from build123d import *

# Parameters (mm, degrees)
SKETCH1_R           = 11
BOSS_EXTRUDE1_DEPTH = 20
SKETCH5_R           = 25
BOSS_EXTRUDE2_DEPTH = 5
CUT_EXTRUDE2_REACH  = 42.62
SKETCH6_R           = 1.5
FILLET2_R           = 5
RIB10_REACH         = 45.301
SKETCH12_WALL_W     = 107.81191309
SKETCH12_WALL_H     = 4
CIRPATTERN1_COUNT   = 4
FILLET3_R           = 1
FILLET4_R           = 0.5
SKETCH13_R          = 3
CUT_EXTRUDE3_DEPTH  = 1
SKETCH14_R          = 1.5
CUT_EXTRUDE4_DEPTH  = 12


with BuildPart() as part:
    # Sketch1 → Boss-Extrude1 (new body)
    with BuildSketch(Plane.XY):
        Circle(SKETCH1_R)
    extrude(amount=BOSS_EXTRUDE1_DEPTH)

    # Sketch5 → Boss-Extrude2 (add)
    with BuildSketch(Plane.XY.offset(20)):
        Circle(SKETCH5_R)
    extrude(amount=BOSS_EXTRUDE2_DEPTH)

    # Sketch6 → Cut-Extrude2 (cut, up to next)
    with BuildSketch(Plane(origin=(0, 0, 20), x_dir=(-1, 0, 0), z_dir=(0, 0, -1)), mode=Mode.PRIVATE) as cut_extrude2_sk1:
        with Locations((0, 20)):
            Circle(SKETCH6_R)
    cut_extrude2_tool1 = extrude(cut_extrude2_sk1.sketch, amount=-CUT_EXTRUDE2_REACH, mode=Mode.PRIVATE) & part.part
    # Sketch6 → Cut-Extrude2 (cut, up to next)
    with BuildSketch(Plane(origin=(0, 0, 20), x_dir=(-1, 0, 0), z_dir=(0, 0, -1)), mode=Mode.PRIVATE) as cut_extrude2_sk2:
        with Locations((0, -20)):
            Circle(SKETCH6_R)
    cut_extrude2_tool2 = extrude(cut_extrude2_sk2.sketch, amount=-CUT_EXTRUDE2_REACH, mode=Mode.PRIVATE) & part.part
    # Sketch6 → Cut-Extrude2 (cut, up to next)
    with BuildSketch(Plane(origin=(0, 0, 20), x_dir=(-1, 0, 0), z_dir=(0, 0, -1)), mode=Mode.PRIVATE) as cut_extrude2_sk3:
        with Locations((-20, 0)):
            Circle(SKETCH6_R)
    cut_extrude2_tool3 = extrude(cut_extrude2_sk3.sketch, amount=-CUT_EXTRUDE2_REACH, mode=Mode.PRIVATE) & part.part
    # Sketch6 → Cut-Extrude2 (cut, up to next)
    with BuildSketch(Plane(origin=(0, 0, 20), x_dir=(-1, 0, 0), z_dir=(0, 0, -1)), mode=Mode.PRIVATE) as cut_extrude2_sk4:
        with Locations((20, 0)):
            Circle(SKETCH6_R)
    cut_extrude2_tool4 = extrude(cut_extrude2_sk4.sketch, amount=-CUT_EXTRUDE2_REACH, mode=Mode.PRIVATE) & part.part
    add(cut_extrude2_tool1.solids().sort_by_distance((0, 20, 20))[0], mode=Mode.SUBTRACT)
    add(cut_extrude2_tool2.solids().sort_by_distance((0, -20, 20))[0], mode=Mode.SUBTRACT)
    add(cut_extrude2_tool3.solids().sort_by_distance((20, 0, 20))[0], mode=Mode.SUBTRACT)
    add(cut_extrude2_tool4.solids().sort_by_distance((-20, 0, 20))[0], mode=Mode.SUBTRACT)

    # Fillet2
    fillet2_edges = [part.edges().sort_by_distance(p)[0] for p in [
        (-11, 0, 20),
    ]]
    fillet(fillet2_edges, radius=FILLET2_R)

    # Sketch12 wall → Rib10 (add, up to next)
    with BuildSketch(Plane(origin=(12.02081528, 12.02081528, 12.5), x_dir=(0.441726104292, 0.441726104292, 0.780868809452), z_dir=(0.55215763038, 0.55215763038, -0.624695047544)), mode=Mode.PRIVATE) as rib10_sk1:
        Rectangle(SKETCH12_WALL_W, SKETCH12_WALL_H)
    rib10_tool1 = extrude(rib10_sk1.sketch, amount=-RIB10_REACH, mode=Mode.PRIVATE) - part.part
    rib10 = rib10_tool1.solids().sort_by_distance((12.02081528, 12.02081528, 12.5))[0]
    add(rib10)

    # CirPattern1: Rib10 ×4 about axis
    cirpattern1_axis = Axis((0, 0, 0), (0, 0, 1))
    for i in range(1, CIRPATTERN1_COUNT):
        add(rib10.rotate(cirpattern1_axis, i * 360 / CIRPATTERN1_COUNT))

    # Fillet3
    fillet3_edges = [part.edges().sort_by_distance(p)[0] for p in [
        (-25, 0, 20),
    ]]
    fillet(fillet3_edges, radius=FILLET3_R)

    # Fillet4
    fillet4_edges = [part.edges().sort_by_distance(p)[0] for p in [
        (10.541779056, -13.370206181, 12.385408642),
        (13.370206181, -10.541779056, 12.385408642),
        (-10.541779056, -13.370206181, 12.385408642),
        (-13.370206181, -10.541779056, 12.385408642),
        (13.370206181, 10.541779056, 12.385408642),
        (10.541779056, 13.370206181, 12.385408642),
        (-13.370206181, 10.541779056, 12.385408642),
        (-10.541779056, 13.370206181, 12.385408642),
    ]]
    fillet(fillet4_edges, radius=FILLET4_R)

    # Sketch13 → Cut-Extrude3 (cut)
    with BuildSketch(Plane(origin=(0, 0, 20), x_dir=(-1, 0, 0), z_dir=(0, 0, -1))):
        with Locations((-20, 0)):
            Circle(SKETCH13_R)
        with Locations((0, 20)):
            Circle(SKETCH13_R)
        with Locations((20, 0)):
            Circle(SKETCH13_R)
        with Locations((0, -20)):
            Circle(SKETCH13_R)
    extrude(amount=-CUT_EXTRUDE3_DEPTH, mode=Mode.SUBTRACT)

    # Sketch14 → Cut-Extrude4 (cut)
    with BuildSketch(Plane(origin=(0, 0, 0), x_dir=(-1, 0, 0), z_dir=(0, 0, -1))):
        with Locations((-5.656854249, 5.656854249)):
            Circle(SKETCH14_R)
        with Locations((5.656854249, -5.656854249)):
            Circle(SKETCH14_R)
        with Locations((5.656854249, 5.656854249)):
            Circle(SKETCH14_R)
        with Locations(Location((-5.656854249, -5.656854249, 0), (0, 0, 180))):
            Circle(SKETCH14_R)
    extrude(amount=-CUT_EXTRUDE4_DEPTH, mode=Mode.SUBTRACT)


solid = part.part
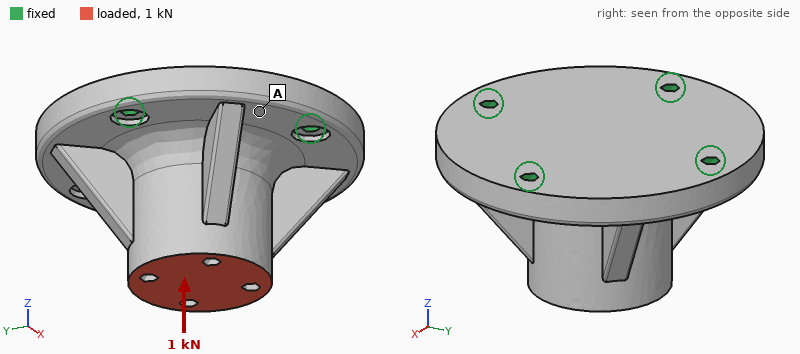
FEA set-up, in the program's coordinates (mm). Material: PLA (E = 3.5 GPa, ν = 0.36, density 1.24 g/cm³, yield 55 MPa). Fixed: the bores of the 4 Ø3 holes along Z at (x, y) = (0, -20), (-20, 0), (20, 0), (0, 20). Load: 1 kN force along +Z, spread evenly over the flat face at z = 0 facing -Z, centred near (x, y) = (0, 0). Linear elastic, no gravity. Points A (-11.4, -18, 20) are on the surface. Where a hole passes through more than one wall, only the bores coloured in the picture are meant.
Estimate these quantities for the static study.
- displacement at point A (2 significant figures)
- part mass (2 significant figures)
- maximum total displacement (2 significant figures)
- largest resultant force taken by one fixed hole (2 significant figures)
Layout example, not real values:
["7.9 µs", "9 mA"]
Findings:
["41 µm", "23 g", "72 µm", "280 N"]
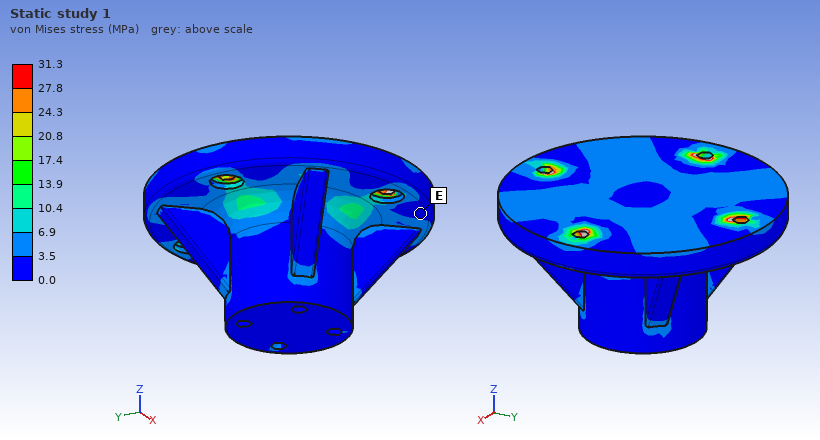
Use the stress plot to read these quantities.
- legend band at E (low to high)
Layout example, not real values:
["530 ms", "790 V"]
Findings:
["0.0 to 3.5 MPa"]
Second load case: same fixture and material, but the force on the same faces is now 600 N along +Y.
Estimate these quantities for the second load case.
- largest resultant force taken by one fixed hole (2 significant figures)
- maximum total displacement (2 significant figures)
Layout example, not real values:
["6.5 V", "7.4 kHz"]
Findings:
["430 N", "0.18 mm"]
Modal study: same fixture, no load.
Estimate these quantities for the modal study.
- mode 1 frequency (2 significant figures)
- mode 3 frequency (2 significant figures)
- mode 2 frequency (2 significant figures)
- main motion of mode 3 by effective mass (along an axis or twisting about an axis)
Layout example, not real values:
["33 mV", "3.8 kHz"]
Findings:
["4400 Hz", "4800 Hz", "4400 Hz", "along Z"]
